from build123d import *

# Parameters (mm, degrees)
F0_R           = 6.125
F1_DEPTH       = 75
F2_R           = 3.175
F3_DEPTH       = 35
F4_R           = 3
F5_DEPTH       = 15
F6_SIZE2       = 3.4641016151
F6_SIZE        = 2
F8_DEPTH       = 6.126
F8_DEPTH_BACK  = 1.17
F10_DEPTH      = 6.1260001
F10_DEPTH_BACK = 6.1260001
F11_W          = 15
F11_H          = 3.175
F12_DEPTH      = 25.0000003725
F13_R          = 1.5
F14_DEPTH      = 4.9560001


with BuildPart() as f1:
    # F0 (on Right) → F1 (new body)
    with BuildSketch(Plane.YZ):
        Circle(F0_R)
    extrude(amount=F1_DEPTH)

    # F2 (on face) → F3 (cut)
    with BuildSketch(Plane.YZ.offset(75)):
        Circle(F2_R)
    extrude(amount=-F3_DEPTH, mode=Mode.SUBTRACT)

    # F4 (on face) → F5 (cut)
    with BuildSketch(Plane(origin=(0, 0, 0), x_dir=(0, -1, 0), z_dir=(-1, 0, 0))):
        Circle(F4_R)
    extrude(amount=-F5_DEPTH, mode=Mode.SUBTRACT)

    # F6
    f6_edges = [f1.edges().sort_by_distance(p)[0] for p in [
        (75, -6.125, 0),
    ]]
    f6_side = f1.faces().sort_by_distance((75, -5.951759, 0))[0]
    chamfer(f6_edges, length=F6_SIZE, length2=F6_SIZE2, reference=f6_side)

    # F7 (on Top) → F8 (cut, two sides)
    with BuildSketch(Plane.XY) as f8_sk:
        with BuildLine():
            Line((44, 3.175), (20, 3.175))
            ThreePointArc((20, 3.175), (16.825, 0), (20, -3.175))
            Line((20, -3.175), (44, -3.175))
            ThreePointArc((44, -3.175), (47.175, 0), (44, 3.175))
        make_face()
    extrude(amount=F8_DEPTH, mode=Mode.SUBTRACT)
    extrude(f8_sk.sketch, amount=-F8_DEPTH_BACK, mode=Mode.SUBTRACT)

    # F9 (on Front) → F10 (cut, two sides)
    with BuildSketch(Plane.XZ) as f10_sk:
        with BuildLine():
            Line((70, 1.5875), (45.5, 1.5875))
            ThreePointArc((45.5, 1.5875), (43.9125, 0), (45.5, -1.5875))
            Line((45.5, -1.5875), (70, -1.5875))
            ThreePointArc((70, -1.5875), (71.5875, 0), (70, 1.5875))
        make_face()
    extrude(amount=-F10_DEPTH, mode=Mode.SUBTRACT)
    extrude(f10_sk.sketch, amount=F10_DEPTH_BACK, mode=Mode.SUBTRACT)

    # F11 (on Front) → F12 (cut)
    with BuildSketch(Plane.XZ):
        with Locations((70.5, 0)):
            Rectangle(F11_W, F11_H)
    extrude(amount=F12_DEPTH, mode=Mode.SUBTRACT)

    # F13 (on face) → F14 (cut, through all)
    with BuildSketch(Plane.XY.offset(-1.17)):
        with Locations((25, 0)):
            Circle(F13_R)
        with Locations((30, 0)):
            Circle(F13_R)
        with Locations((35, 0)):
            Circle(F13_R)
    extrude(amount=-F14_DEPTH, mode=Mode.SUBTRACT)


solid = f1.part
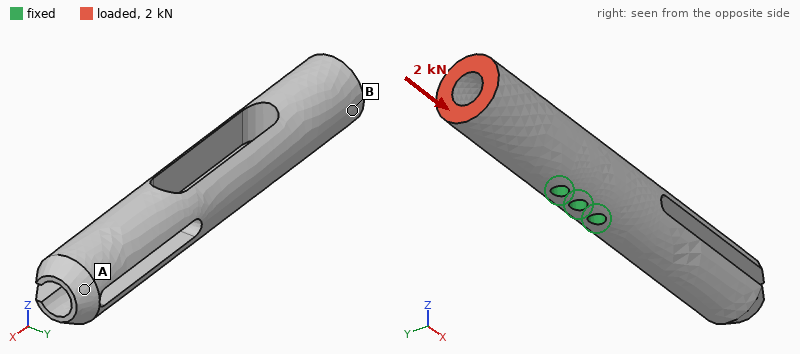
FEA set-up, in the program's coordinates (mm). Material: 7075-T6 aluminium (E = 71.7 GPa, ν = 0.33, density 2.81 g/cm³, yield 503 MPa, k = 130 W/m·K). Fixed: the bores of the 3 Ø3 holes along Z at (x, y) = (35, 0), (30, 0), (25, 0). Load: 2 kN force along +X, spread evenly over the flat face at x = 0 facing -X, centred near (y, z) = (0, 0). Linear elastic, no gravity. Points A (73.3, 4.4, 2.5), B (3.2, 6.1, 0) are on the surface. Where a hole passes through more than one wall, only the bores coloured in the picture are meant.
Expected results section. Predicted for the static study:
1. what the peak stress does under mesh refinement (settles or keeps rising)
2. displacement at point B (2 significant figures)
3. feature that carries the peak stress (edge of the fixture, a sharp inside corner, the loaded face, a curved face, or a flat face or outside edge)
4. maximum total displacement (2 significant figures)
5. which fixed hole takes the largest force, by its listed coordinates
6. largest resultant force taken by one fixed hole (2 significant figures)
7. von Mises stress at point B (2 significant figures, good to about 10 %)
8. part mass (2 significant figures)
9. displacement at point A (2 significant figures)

keeps rising
30 µm
edge of the fixture
39 µm
(25, 0)
1.2 kN
22 MPa
15 g
14 µm
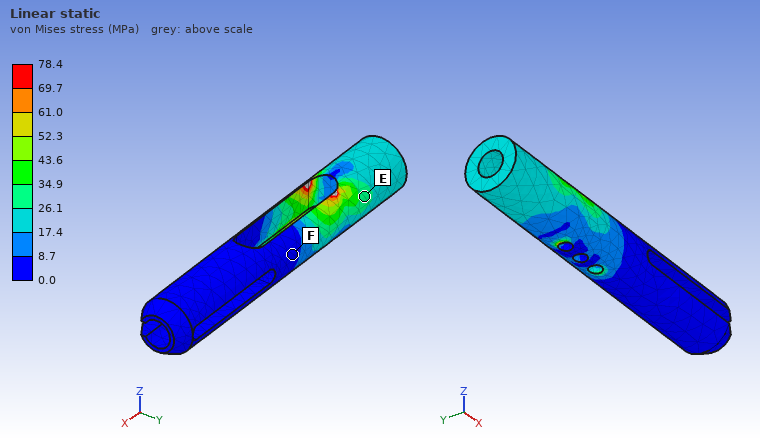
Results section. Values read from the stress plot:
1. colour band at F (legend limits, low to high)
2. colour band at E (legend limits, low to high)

0.0 to 8.7 MPa
26.1 to 34.9 MPa
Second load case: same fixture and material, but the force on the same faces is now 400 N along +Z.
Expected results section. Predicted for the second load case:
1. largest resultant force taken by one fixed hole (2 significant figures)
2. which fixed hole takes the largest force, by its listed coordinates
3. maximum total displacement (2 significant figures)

1.1 kN
(25, 0)
80 µm
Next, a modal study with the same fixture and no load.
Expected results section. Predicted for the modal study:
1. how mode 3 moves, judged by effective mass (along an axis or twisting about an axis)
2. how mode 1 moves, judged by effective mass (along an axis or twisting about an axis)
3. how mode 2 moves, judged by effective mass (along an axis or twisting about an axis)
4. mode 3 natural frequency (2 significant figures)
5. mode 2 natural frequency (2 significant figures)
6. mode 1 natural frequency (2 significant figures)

along Z
along Z
along Y
8400 Hz
4600 Hz
3000 Hz
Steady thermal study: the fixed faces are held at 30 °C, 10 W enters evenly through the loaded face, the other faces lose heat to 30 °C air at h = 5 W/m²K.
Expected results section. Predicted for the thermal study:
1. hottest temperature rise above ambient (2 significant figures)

24 K
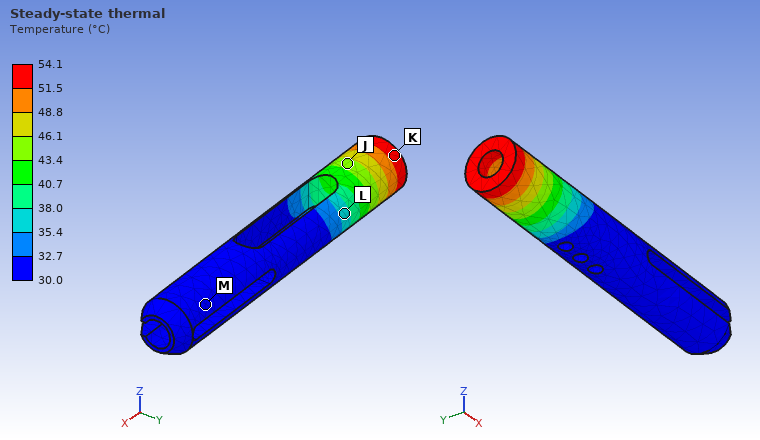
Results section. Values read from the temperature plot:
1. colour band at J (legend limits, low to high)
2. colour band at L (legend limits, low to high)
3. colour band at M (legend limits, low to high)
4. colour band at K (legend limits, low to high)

43.4 to 46.1 °C
35.4 to 38.0 °C
30.0 to 32.7 °C
51.5 to 54.1 °C
